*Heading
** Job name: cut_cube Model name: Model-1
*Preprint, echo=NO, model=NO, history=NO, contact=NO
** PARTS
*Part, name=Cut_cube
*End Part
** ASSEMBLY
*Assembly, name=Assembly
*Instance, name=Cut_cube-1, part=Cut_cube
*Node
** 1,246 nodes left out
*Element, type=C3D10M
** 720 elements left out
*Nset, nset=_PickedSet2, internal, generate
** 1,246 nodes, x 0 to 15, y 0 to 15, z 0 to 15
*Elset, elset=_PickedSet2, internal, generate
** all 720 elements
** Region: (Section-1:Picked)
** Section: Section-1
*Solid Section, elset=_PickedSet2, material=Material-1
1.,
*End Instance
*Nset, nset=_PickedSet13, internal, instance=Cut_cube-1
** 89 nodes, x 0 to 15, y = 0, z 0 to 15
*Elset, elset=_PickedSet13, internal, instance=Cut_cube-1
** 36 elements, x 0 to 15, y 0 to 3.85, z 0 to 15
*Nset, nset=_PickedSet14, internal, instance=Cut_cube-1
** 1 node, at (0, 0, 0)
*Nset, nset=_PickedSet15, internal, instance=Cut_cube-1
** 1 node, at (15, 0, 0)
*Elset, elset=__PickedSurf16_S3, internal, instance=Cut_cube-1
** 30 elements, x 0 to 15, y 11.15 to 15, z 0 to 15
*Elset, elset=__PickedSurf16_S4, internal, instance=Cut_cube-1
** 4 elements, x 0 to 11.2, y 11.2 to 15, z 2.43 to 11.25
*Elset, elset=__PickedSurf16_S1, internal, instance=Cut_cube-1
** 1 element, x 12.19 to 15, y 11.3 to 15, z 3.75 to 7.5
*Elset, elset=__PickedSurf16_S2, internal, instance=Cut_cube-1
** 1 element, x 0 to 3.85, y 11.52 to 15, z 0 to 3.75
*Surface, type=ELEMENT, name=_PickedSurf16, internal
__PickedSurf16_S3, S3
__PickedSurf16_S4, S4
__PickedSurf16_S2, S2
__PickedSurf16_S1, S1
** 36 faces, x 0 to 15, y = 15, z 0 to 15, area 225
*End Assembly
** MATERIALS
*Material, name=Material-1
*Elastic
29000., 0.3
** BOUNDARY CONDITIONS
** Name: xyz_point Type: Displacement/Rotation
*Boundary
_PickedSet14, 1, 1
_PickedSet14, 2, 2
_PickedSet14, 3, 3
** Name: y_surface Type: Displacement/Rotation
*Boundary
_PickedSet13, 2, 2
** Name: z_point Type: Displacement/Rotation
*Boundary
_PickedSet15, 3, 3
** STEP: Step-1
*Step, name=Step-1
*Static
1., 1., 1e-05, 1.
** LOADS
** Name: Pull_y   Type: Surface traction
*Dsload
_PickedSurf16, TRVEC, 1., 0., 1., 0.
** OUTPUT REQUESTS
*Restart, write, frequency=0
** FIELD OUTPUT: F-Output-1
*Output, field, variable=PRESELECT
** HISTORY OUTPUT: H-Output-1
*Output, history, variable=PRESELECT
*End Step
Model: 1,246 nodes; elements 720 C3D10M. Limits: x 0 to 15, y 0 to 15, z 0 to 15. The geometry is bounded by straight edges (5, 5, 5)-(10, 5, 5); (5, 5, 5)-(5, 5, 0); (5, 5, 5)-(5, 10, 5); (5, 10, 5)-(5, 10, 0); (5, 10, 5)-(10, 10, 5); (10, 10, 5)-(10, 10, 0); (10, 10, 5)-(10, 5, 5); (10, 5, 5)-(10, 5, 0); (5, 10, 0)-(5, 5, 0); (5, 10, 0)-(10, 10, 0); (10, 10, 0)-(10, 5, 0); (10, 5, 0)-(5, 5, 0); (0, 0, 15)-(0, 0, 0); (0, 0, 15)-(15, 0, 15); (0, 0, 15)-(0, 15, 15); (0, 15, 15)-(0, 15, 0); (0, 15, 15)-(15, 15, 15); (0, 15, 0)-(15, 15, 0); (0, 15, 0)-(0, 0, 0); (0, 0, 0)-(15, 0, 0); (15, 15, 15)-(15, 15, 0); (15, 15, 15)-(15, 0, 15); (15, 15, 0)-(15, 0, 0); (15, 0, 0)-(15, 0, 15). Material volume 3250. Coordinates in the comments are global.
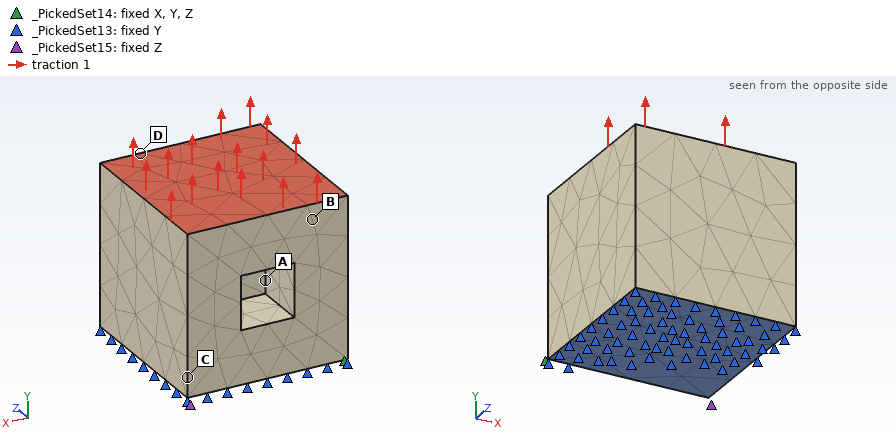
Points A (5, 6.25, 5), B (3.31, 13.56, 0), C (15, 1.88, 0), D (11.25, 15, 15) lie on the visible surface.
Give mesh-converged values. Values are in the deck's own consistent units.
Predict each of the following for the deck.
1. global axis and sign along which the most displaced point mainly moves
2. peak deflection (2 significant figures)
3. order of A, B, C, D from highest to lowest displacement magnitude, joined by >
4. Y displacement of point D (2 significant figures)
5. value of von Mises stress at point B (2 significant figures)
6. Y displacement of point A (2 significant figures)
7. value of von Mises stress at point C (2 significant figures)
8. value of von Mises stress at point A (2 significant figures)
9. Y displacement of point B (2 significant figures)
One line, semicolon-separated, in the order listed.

+Y; 8.3e-04; B > D > A > C; 4.8e-04; 1.2; 2.4e-04; 1.4; 1.5; 6.4e-04
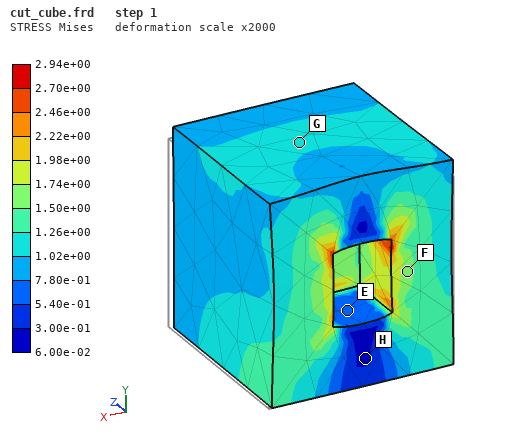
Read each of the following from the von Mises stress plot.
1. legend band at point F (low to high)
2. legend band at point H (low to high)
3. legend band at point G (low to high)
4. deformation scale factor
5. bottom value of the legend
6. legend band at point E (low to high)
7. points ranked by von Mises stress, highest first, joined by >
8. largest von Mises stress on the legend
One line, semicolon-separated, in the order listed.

1.50e+00 to 1.74e+00; 6.00e-02 to 3.00e-01; 1.02e+00 to 1.26e+00; 2000; 6.00e-02; 5.40e-01 to 7.80e-01; F > G > E > H; 2.94e+00
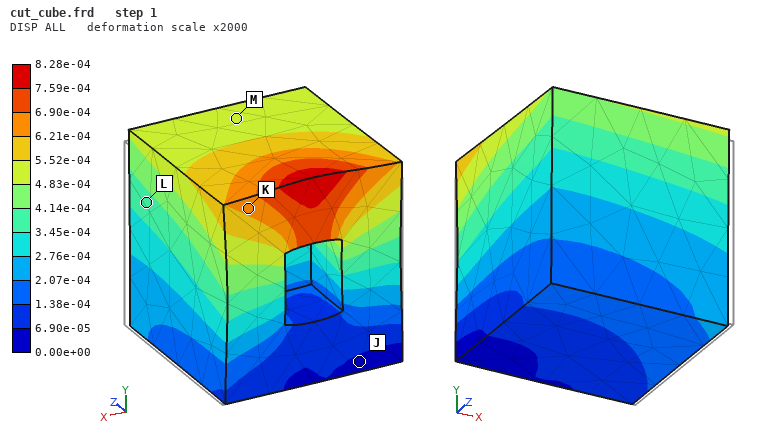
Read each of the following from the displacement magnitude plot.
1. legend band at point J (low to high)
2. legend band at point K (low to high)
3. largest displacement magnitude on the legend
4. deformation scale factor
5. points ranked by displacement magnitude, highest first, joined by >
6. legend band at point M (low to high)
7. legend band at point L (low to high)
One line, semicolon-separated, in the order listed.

0.00e+00 to 6.90e-05; 6.21e-04 to 6.90e-04; 8.28e-04; 2000; K > M > L > J; 4.83e-04 to 5.52e-04; 3.45e-04 to 4.14e-04
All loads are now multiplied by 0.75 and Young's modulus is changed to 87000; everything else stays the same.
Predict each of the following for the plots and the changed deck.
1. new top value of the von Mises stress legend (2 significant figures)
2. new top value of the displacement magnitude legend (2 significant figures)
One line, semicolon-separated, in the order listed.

2.2; 2.1e-04
